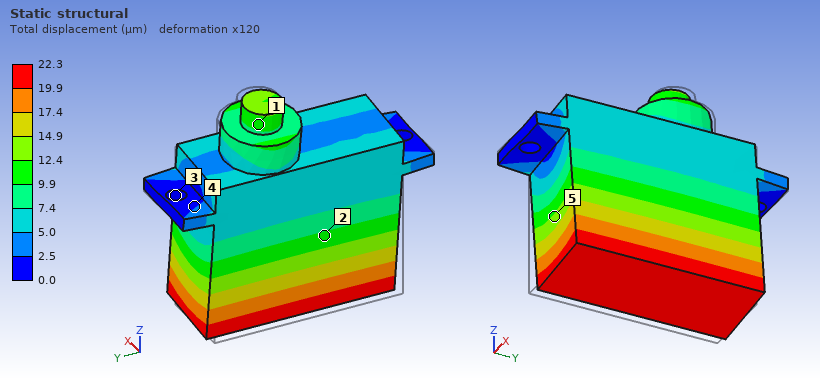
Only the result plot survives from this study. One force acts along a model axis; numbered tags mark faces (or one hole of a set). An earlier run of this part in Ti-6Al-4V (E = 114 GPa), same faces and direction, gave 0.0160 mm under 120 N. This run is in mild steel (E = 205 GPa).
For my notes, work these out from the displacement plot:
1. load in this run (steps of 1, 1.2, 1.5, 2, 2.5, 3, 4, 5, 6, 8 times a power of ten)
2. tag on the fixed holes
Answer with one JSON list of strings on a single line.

["300 N", "3"]
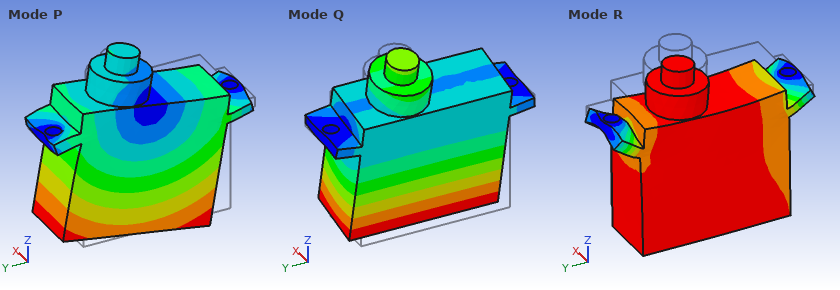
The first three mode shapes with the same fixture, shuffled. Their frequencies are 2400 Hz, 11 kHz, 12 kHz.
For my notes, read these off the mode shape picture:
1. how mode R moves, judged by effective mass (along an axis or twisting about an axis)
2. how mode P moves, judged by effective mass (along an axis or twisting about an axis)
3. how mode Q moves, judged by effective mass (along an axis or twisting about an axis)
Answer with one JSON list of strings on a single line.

["along Z", "along Y", "along X"]
